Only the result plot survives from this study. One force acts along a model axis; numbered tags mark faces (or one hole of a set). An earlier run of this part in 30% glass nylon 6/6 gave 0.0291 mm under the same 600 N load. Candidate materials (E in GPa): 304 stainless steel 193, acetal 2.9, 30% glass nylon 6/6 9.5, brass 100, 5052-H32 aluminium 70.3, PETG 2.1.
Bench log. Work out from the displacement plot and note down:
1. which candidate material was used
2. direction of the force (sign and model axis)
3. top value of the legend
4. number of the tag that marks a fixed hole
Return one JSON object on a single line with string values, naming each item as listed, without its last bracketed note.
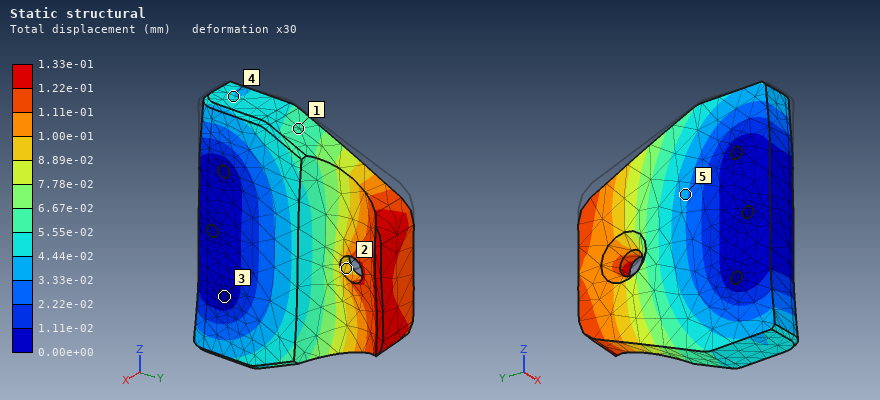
{"which candidate material was used": "PETG", "direction of the force": "-Z", "top value of the legend": "1.33e-01 mm", "number of the tag that marks a fixed hole": "3"}
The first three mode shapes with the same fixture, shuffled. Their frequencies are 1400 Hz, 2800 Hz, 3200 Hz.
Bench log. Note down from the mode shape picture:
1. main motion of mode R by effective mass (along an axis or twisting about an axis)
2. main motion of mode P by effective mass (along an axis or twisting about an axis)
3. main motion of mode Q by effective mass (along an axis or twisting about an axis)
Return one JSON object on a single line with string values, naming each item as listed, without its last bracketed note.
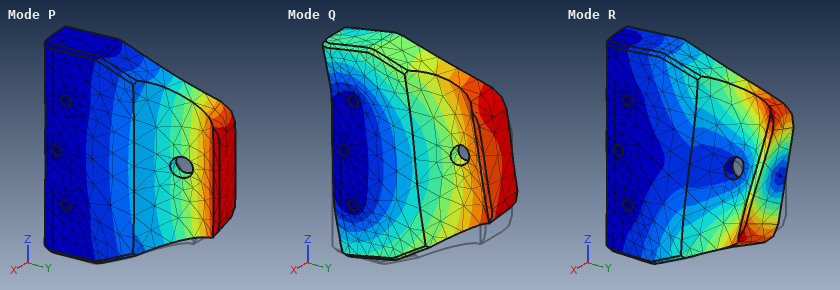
{"main motion of mode R by effective mass": "twisting about Y", "main motion of mode P by effective mass": "along X", "main motion of mode Q by effective mass": "along Z"}
